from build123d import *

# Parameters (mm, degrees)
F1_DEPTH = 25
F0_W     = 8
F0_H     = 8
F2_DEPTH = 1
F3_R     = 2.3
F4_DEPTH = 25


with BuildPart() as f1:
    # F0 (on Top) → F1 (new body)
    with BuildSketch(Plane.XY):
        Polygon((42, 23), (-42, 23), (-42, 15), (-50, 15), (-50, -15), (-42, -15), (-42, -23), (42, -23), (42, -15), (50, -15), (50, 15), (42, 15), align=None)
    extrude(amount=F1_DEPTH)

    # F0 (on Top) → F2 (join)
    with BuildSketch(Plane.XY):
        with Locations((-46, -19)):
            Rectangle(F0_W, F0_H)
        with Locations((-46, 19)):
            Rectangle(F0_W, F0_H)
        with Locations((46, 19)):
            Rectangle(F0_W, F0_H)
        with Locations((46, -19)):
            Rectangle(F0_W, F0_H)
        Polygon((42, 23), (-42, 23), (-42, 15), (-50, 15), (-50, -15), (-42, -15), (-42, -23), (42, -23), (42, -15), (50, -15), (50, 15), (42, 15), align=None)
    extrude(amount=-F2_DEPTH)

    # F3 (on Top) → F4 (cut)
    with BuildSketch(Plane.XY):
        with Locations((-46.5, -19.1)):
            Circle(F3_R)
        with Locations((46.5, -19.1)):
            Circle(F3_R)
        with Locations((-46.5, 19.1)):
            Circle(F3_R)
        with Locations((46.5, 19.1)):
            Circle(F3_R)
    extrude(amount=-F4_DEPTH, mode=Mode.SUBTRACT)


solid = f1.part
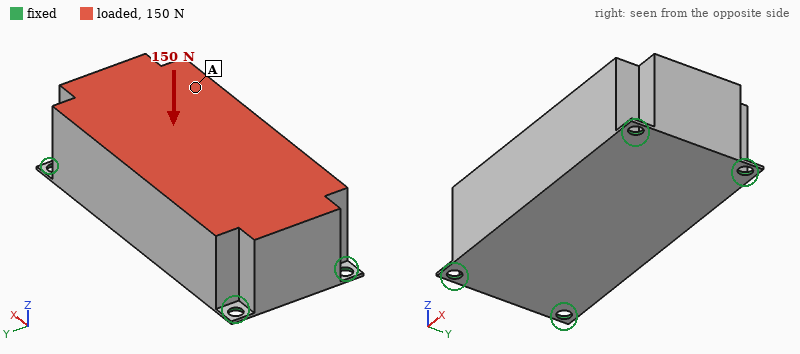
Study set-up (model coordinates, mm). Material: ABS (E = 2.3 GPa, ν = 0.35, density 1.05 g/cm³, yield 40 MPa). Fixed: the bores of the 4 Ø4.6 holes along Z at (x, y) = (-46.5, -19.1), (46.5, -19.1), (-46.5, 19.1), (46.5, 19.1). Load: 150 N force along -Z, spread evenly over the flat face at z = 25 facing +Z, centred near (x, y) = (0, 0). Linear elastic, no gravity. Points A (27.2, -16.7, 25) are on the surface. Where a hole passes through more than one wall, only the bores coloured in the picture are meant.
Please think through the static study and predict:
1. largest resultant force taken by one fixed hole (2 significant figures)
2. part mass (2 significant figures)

44 N
120 g
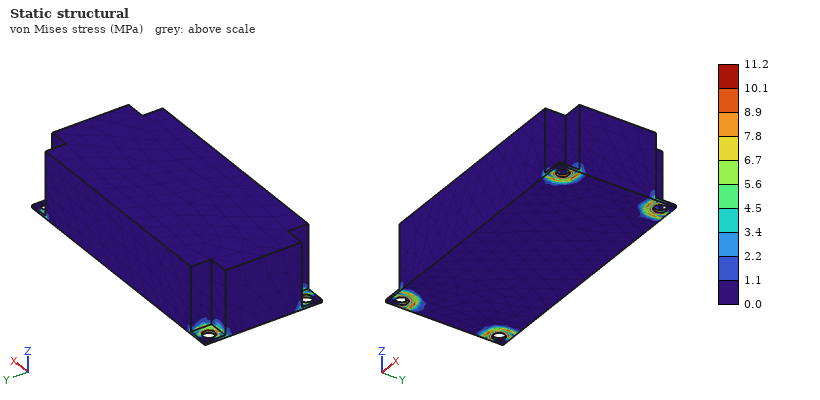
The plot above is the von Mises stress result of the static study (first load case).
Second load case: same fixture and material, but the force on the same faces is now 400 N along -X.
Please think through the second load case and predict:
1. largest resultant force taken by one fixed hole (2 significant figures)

120 N
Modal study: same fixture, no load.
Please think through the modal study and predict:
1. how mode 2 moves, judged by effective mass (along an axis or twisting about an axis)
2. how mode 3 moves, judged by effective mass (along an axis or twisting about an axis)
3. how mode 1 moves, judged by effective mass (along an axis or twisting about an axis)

along Z
along X
along Y
